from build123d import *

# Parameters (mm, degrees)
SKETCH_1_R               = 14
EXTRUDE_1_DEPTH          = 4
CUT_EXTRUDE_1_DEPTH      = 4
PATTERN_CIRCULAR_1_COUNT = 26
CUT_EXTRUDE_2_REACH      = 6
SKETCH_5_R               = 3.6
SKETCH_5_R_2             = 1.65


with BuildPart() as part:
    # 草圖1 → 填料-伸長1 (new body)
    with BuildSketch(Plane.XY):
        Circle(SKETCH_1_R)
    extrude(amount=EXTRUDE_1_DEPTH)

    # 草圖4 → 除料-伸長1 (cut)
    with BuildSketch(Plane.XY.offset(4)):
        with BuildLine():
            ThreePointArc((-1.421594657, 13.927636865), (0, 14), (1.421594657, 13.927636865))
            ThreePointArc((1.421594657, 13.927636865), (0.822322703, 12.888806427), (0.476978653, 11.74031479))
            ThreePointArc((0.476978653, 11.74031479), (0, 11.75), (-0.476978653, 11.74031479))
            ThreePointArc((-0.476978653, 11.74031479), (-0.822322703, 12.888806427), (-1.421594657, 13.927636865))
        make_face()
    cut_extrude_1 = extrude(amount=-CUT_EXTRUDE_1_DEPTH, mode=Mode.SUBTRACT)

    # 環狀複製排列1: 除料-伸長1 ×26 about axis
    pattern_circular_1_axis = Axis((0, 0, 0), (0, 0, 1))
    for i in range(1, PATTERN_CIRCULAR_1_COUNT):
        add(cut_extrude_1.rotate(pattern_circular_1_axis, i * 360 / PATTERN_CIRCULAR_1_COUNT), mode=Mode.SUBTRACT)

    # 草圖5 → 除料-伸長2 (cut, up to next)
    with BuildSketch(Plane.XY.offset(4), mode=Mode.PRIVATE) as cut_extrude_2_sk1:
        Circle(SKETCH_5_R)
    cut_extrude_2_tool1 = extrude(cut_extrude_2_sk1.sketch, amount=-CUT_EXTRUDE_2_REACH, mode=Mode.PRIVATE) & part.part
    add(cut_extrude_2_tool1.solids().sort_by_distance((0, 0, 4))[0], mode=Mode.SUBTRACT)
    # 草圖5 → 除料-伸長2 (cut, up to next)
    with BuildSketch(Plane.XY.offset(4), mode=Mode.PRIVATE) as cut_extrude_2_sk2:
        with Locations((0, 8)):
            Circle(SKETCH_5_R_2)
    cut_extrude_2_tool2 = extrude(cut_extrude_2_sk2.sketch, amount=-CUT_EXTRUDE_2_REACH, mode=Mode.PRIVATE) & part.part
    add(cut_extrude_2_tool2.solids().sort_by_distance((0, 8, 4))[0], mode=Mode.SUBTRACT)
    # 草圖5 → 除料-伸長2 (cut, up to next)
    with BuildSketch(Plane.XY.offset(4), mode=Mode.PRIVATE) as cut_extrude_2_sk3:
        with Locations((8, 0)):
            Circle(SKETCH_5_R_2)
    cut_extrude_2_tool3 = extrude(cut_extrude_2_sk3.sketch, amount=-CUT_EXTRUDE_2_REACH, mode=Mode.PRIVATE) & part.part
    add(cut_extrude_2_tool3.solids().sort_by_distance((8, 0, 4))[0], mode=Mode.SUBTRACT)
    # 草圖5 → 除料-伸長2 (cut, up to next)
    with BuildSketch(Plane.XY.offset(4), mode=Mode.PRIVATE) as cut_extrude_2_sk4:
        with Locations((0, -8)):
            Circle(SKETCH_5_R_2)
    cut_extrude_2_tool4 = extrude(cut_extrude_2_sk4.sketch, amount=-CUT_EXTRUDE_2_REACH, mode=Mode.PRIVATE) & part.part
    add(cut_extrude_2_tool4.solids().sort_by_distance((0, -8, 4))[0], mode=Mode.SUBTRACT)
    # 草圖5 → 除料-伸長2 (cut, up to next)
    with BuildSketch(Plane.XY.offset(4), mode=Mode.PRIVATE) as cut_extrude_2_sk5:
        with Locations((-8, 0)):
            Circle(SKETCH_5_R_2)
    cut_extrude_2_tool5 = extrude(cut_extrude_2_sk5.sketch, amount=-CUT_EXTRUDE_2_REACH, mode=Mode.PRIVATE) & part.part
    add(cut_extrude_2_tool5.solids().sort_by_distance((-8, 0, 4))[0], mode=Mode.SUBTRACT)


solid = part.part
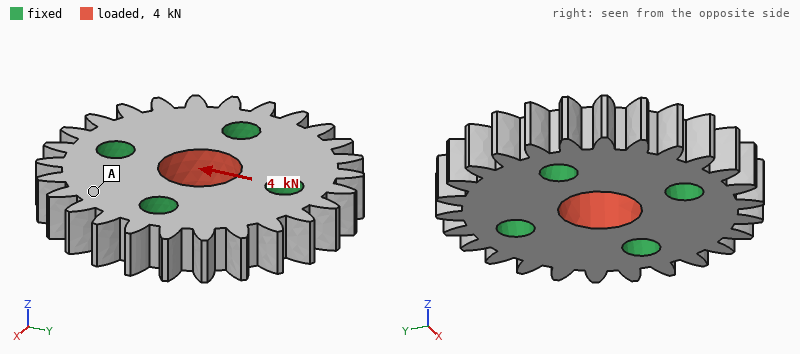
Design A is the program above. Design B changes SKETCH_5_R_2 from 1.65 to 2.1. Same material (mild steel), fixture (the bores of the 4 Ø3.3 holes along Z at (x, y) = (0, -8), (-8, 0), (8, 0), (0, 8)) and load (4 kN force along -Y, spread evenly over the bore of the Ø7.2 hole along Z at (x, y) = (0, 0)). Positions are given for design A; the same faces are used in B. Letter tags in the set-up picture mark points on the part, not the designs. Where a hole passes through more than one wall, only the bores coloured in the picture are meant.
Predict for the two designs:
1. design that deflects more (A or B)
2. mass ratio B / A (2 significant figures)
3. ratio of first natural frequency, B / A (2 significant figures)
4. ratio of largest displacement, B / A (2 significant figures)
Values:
A
0.95
1.1
0.86
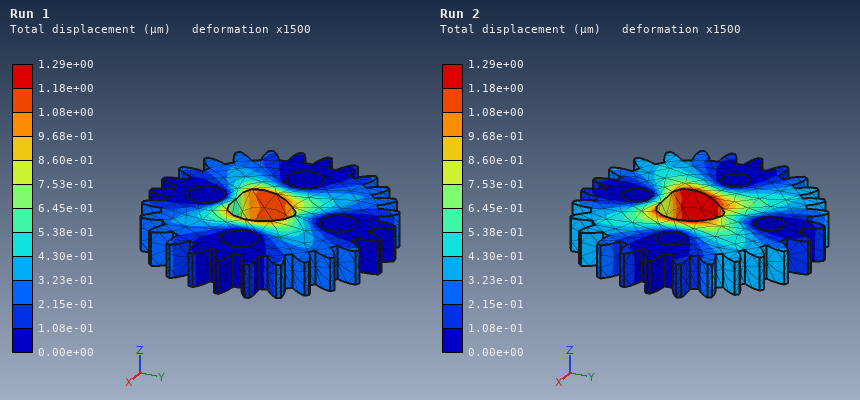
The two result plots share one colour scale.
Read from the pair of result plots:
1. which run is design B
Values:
Run 1
